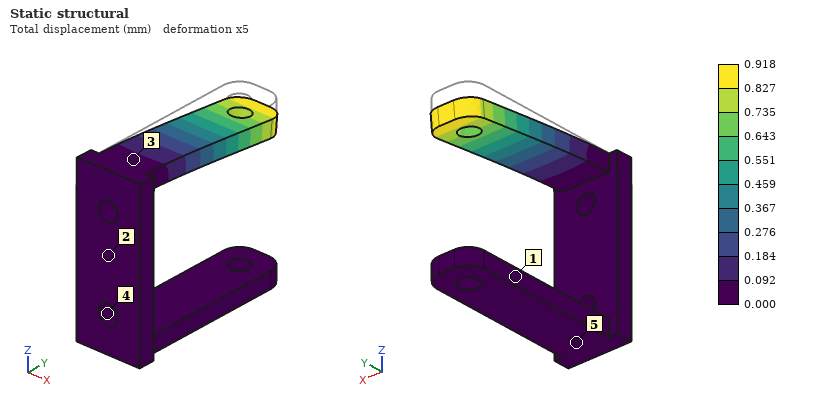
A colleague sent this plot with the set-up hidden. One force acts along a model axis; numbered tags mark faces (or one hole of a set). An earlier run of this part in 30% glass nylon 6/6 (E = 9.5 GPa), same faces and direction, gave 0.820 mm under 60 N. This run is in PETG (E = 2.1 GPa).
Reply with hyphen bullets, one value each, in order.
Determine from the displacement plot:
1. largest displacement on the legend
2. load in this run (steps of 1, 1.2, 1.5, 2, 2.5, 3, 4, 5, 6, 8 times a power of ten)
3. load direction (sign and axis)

- 0.918 mm
- 15 N
- -Z
